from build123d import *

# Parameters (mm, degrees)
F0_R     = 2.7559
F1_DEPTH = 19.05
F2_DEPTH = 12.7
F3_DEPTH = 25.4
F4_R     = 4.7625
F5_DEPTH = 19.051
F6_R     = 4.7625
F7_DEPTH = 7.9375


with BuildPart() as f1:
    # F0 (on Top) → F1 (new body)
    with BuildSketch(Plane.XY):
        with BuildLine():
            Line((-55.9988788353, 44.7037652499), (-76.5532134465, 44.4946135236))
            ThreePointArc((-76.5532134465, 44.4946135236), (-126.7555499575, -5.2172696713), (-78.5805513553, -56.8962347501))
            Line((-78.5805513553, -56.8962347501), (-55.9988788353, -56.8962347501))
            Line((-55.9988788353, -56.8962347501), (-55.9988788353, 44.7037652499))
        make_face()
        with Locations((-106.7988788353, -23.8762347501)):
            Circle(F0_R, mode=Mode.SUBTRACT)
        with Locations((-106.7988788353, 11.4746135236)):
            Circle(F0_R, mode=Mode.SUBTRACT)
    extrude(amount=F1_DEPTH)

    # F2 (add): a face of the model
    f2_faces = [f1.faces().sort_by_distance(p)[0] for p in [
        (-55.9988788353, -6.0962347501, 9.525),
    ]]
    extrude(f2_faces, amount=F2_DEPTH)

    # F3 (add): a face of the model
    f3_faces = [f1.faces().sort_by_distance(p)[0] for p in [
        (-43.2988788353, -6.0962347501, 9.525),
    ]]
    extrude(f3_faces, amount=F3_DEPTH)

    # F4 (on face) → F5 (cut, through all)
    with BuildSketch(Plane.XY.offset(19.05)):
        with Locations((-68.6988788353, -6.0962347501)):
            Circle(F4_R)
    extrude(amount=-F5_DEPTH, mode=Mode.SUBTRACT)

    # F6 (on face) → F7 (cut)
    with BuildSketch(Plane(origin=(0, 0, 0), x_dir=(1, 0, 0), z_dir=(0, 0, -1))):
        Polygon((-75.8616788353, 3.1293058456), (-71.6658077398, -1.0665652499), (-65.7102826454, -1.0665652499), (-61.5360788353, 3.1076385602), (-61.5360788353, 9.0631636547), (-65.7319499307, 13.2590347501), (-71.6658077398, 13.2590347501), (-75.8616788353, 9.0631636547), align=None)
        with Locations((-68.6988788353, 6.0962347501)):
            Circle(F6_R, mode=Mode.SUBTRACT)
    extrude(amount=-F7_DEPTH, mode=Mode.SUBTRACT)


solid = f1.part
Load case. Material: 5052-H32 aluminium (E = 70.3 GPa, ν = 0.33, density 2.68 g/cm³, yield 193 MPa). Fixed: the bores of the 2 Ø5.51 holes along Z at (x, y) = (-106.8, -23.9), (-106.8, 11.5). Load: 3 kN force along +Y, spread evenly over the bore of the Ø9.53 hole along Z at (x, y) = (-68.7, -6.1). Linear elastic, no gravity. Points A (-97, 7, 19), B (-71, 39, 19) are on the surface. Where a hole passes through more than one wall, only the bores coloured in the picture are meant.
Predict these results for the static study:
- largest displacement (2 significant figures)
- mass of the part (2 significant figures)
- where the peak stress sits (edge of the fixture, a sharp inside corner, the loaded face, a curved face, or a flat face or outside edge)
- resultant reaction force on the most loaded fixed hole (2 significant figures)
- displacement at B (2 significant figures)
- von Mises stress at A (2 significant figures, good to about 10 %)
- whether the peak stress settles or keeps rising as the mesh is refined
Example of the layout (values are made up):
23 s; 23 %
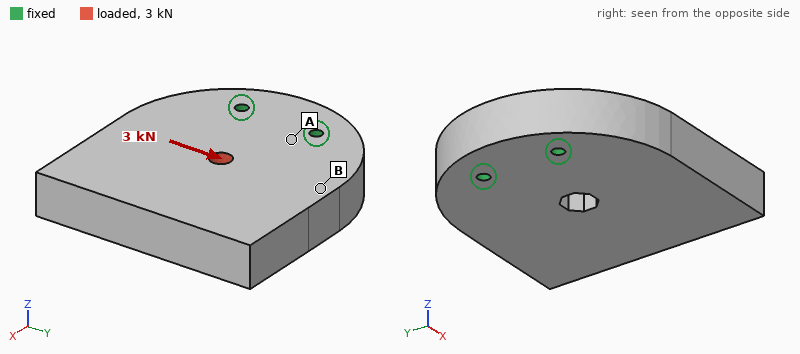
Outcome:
16 µm; 500 g; edge of the fixture; 3.3 kN; 9.2 µm; 9.2 MPa; keeps rising
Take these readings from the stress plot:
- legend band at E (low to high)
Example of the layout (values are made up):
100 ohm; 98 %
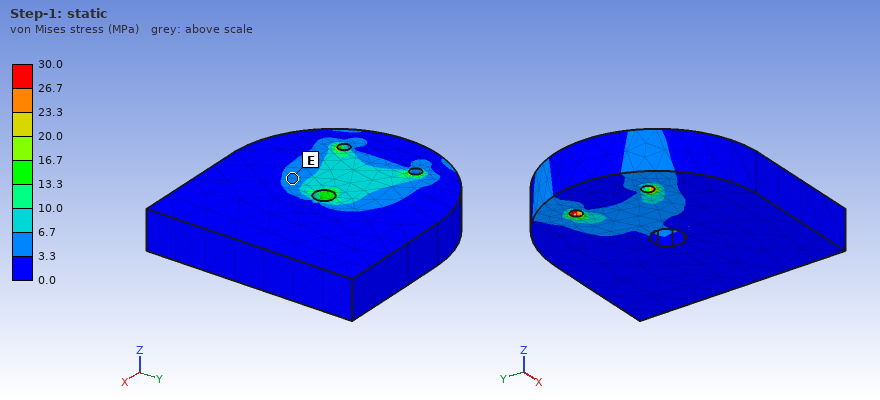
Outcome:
3.3 to 6.7 MPa
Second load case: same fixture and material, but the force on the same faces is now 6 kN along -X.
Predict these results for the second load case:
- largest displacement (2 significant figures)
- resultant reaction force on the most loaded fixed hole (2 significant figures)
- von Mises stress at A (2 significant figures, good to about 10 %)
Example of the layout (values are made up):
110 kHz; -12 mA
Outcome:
23 µm; 3.1 kN; 12 MPa
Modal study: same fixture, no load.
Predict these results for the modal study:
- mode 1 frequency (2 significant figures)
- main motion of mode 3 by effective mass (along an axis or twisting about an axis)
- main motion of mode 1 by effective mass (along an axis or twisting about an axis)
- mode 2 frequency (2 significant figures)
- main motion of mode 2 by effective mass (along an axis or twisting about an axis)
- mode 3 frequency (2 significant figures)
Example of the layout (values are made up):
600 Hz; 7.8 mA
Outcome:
1600 Hz; along Y; along Z; 3100 Hz; twisting about X; 3500 Hz
